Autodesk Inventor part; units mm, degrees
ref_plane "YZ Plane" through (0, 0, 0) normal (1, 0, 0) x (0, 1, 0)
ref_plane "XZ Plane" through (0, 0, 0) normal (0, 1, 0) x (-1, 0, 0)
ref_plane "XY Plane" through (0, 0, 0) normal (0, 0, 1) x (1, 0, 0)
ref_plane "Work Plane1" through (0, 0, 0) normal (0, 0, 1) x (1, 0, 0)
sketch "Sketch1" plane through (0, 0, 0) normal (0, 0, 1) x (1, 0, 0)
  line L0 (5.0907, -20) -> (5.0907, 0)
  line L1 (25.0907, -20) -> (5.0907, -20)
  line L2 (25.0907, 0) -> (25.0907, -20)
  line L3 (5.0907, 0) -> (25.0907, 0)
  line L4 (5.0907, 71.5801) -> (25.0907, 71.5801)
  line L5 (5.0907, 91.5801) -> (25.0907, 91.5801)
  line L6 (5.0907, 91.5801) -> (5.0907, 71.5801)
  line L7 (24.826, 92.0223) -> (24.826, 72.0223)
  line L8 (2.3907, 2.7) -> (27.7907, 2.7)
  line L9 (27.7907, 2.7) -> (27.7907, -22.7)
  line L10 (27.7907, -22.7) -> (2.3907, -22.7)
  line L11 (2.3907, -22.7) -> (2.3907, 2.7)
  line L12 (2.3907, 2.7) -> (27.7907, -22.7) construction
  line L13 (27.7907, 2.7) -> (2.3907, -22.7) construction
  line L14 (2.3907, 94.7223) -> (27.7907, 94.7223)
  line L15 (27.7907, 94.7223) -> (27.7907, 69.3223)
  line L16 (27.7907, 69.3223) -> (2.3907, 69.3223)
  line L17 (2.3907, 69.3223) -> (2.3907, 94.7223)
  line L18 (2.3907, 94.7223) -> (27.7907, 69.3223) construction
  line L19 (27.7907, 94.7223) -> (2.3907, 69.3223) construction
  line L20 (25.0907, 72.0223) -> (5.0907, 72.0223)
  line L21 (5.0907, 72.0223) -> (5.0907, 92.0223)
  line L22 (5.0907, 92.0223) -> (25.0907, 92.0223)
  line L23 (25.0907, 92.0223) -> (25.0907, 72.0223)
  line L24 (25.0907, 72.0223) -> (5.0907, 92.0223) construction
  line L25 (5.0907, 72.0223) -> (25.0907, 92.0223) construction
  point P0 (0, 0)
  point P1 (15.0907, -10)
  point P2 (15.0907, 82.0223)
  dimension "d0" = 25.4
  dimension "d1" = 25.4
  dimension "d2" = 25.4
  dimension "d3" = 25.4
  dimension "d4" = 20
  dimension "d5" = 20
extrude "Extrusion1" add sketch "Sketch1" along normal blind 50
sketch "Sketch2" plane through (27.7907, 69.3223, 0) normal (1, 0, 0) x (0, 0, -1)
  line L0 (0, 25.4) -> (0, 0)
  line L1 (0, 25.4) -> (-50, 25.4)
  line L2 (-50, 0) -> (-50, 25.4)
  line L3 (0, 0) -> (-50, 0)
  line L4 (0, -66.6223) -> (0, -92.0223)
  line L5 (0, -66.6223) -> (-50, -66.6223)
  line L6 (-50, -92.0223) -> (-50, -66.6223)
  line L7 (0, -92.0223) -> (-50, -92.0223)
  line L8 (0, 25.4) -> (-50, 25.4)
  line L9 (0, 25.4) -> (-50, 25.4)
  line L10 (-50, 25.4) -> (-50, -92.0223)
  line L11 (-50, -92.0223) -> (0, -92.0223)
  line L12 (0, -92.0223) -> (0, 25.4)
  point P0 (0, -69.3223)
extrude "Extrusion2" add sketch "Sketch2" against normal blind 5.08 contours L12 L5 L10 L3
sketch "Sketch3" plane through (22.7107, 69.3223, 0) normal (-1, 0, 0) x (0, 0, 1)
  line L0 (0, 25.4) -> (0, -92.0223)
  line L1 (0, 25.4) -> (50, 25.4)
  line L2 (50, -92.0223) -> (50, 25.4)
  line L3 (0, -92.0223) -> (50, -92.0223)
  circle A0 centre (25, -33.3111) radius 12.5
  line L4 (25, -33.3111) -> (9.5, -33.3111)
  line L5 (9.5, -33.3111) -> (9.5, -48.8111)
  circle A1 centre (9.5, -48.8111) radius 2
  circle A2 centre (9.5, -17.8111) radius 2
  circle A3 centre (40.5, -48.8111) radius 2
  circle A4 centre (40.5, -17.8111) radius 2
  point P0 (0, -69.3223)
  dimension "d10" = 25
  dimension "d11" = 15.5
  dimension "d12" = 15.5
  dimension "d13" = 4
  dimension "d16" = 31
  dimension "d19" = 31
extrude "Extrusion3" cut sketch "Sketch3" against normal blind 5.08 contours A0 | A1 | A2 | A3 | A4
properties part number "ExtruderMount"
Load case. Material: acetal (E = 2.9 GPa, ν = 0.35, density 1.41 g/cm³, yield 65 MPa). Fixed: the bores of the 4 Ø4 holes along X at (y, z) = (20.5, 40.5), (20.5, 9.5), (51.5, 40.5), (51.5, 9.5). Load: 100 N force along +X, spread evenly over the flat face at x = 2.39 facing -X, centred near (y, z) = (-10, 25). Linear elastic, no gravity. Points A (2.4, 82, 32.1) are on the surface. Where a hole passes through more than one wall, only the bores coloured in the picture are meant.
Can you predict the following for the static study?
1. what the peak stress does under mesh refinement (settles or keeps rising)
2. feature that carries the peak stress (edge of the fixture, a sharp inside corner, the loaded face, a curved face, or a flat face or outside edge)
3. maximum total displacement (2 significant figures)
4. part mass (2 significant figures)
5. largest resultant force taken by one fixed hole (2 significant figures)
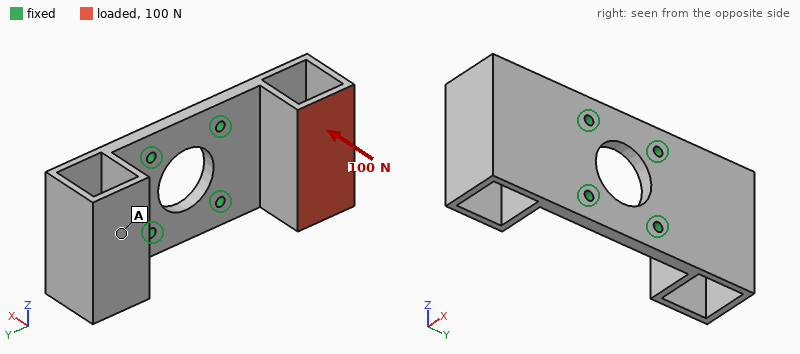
keeps rising
edge of the fixture
1.5 mm
55 g
58 N
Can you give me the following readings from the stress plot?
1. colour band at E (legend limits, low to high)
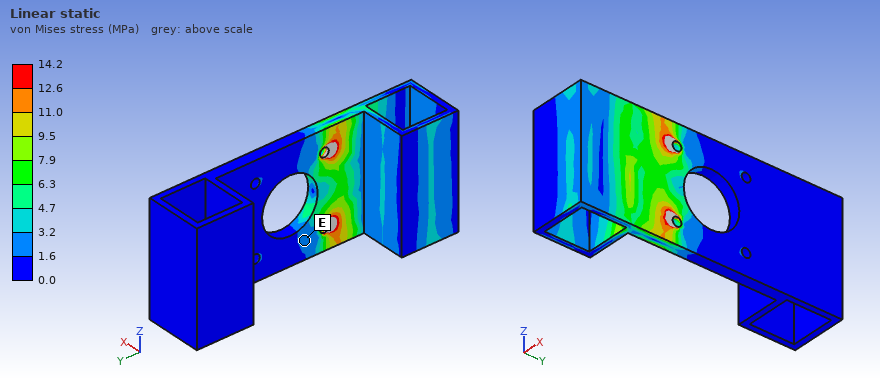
1.6 to 3.2 MPa
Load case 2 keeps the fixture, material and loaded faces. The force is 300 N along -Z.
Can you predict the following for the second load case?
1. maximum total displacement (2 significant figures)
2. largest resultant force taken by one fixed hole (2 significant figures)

1.1 mm
340 N
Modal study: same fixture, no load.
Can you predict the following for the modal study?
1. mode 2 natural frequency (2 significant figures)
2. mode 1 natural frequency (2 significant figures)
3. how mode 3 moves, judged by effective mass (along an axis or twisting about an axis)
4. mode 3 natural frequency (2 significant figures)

340 Hz
330 Hz
along Z
940 Hz
